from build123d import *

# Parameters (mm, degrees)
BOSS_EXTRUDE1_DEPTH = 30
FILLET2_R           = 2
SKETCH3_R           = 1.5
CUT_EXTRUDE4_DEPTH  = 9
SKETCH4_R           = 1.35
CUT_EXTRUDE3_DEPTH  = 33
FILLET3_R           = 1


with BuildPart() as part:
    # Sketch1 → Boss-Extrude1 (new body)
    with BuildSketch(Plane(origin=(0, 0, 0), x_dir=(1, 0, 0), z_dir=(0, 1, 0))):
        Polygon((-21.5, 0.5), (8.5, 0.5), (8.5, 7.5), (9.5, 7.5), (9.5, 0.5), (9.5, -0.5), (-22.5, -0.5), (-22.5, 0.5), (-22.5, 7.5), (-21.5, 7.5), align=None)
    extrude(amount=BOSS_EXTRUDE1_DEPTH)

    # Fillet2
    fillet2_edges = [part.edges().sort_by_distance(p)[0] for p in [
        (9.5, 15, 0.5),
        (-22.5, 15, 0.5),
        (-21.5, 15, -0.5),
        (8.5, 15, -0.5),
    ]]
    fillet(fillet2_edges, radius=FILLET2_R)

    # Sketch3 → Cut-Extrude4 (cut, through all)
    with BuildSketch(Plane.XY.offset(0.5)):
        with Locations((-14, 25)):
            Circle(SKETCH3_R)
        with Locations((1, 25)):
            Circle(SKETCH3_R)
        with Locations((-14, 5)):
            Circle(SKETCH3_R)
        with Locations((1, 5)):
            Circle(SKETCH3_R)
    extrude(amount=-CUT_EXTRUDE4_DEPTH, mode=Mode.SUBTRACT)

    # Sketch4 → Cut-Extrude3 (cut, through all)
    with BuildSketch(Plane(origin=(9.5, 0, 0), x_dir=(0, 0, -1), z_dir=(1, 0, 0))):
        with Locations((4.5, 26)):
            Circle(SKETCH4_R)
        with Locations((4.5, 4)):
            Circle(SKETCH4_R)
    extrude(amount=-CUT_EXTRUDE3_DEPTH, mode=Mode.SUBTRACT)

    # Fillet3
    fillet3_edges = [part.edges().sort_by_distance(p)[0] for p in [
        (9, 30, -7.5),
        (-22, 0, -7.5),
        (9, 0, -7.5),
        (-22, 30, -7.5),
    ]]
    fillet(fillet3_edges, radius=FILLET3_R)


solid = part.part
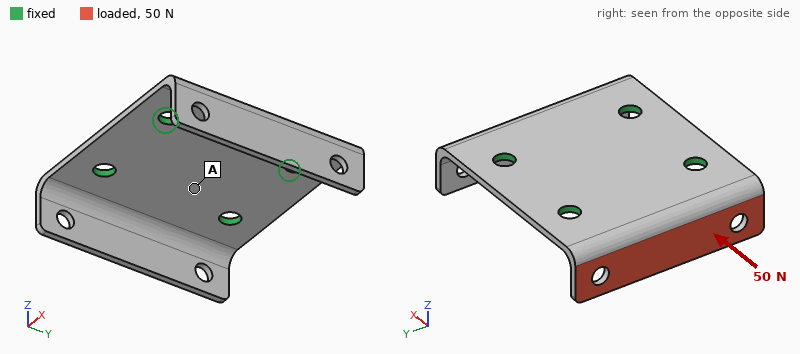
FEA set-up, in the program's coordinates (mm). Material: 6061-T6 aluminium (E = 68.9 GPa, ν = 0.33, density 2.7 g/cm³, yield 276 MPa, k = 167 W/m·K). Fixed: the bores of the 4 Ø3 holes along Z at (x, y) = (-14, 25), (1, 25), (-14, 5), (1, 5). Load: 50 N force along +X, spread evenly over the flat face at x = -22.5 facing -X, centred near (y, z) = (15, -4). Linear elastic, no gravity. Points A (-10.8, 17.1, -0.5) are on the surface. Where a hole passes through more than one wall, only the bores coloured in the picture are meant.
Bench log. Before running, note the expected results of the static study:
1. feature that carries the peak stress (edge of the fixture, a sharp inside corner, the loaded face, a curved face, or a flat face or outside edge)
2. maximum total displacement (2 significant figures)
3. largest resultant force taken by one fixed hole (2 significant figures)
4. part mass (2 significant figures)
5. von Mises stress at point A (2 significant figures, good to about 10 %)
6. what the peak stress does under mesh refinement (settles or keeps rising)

edge of the fixture
78 µm
20 N
3.6 g
9.0 MPa
keeps rising
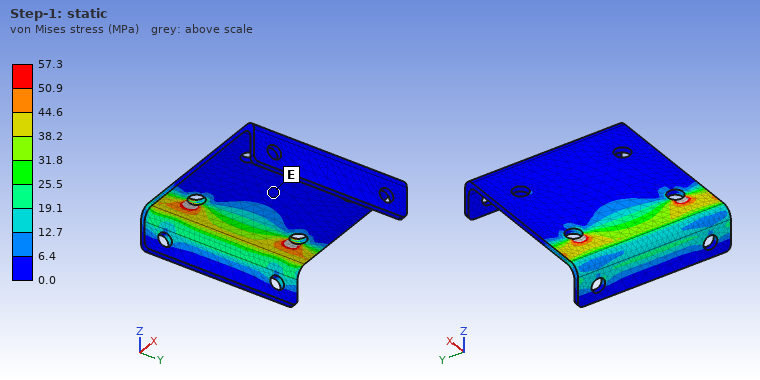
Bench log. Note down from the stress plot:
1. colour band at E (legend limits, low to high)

0.0 to 6.4 MPa
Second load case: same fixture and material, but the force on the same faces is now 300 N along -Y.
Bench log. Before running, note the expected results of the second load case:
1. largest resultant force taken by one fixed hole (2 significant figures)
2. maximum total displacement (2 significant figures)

190 N
0.12 mm
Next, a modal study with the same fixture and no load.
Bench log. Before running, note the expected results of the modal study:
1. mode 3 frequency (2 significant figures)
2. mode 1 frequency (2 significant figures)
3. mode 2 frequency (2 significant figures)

7900 Hz
5200 Hz
5200 Hz
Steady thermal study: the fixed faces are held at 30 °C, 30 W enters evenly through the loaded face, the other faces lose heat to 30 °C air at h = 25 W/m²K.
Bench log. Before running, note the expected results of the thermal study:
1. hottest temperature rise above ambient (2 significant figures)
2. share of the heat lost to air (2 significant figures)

74 K
3.1 %
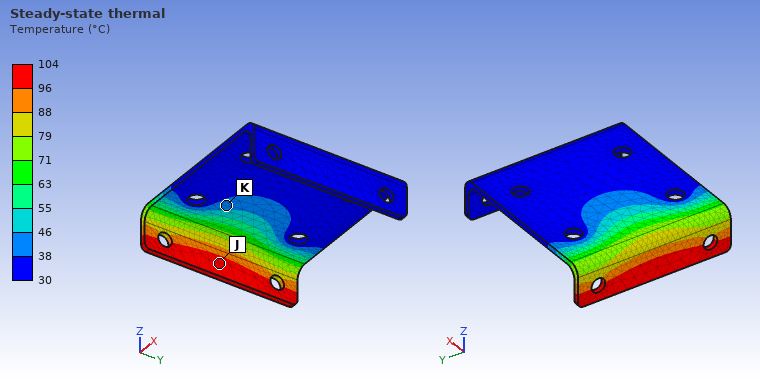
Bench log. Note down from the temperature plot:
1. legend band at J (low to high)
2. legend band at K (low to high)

96 to 104 °C
38 to 46 °C
